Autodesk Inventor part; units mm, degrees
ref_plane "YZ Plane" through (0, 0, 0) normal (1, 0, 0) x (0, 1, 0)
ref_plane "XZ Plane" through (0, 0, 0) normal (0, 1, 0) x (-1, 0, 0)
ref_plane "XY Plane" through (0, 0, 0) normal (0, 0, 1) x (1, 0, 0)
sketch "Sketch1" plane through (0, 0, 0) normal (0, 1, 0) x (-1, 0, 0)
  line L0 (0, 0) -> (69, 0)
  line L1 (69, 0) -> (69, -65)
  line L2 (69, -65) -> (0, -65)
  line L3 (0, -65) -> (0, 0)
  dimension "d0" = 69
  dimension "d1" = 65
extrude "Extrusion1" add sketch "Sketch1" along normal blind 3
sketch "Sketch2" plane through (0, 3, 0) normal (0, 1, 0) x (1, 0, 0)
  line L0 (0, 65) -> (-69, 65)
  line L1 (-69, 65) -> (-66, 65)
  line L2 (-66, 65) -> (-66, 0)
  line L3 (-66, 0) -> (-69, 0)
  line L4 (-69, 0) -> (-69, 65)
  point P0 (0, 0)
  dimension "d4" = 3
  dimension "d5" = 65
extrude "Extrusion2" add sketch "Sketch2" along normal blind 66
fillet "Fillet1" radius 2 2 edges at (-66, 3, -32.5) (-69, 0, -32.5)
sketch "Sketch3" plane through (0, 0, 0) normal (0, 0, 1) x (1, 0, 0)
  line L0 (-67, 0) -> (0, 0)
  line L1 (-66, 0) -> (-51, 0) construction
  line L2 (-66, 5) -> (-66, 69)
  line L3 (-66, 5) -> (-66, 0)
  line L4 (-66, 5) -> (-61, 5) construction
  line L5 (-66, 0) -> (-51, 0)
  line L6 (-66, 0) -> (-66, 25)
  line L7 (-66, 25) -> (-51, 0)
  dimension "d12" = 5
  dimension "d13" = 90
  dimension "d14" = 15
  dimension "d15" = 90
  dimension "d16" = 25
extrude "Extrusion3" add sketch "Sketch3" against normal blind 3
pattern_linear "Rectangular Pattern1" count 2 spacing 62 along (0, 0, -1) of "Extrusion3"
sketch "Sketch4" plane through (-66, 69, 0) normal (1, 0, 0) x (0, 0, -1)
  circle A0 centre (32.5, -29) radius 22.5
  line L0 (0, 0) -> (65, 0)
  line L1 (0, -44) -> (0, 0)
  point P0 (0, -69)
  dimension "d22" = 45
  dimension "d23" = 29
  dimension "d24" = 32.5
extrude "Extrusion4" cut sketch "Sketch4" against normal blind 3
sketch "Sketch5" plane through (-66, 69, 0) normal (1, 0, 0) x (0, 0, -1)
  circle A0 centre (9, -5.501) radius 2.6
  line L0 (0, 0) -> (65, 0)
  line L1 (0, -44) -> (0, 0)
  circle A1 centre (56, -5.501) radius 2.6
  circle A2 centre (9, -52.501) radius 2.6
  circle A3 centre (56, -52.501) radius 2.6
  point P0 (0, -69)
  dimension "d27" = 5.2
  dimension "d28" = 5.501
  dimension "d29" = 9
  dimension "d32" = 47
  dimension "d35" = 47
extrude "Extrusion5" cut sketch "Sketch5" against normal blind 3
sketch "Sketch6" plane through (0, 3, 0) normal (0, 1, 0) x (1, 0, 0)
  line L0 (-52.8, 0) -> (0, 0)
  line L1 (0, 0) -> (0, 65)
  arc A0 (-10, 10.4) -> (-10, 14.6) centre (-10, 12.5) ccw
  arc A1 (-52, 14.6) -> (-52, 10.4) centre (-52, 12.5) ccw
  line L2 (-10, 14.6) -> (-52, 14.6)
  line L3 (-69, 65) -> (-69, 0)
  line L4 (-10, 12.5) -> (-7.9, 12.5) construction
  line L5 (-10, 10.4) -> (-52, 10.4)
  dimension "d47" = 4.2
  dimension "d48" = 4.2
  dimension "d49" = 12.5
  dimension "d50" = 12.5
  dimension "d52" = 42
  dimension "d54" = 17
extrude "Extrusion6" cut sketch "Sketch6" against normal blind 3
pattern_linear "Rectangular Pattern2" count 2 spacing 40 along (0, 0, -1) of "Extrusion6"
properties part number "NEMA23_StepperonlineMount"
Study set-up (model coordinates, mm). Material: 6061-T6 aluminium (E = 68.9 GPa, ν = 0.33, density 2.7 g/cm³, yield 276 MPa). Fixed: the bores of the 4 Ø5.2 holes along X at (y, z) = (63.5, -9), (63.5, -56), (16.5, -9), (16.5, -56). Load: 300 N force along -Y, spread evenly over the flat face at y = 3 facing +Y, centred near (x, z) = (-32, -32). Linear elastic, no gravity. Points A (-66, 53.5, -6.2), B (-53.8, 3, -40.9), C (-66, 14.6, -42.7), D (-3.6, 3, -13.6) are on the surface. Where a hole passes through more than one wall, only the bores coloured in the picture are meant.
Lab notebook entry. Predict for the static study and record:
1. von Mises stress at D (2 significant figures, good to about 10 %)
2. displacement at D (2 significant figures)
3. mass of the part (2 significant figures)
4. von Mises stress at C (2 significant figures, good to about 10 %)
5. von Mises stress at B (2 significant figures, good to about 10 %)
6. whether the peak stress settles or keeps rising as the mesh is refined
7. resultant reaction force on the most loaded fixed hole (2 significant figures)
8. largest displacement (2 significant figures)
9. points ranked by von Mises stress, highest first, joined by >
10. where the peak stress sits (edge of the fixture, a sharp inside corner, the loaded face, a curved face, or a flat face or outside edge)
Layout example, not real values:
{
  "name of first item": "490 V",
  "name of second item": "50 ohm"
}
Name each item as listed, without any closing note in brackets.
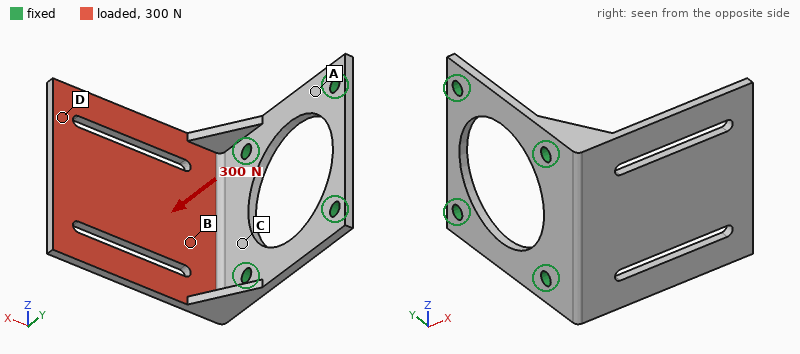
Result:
{
  "von Mises stress at D": "20 MPa",
  "displacement at D": "1.2 mm",
  "mass of the part": "57 g",
  "von Mises stress at C": "37 MPa",
  "von Mises stress at B": "56 MPa",
  "whether the peak stress settles or keeps rising as the mesh is refined": "keeps rising",
  "resultant reaction force on the most loaded fixed hole": "180 N",
  "largest displacement": "1.3 mm",
  "points ranked by von Mises stress, highest first, joined by >": "B > C > D > A",
  "where the peak stress sits": "edge of the fixture"
}
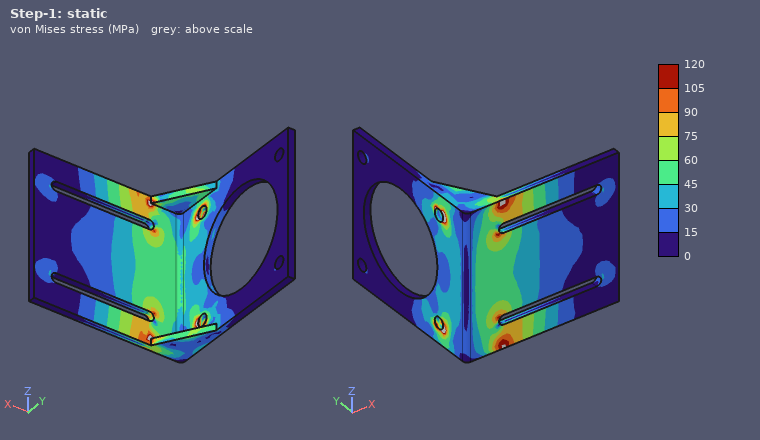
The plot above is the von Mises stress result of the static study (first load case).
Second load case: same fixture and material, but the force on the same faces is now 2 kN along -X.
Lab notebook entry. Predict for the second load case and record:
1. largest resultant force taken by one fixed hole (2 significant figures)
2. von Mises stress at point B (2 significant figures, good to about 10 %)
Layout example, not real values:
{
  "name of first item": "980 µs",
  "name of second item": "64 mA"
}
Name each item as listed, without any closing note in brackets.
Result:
{
  "largest resultant force taken by one fixed hole": "1.0 kN",
  "von Mises stress at point B": "28 MPa"
}
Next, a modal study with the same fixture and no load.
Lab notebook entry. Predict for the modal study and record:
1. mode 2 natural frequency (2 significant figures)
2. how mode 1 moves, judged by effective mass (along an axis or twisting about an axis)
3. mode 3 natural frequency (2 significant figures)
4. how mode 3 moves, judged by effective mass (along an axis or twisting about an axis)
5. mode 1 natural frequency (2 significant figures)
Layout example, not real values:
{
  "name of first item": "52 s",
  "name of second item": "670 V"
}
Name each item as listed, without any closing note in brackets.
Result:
{
  "mode 2 natural frequency": "1400 Hz",
  "how mode 1 moves, judged by effective mass": "along Y",
  "mode 3 natural frequency": "2200 Hz",
  "how mode 3 moves, judged by effective mass": "along Z",
  "mode 1 natural frequency": "540 Hz"
}
